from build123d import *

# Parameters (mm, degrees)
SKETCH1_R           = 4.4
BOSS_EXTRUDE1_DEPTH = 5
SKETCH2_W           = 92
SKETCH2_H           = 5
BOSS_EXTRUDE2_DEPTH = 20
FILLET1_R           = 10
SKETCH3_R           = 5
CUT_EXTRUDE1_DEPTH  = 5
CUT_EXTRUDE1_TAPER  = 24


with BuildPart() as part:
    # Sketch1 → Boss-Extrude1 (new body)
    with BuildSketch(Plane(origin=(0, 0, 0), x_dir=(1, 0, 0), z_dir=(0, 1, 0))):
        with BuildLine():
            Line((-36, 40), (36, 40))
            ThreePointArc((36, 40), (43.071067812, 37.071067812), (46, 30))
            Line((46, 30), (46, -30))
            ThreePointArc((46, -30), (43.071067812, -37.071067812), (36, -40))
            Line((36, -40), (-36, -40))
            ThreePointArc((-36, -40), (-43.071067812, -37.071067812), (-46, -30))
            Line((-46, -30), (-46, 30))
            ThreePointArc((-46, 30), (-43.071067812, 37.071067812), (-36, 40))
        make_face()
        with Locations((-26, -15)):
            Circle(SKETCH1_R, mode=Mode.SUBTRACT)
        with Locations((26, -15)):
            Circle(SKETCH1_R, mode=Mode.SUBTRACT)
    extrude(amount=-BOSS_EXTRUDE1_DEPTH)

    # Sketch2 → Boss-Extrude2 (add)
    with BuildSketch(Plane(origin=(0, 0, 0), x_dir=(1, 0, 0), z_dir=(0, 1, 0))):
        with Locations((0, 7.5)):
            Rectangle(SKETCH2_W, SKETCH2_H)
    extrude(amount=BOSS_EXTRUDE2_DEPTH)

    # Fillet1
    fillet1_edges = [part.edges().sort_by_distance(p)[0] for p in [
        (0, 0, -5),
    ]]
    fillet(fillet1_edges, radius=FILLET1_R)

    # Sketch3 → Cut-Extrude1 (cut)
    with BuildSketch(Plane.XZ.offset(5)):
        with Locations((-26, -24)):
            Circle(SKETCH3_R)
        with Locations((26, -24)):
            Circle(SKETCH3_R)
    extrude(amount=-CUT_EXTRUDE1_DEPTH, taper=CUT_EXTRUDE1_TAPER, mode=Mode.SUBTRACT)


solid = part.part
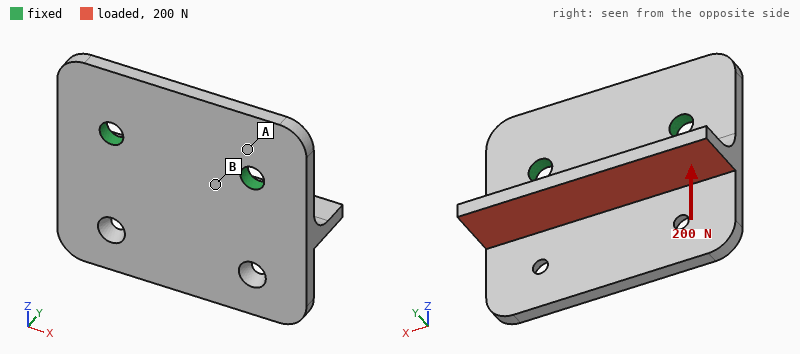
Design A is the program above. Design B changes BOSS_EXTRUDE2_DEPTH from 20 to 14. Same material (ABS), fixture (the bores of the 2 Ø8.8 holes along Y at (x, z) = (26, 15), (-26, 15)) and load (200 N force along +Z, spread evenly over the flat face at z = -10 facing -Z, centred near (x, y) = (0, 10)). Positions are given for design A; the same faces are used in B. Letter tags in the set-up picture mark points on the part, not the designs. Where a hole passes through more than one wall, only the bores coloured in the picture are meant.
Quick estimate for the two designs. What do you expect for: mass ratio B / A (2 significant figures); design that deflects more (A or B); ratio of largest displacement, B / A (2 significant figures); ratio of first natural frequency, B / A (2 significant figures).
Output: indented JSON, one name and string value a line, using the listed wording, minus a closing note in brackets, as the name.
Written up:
{
  "mass ratio B / A": "0.94",
  "design that deflects more": "A",
  "ratio of largest displacement, B / A": "0.76",
  "ratio of first natural frequency, B / A": "1.0"
}
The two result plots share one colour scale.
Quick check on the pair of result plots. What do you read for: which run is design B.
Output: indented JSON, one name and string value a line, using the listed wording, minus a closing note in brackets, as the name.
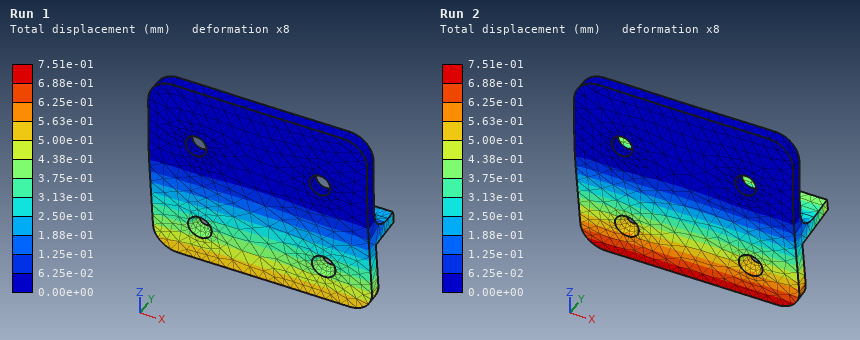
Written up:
{
  "which run is design B": "Run 1"
}
